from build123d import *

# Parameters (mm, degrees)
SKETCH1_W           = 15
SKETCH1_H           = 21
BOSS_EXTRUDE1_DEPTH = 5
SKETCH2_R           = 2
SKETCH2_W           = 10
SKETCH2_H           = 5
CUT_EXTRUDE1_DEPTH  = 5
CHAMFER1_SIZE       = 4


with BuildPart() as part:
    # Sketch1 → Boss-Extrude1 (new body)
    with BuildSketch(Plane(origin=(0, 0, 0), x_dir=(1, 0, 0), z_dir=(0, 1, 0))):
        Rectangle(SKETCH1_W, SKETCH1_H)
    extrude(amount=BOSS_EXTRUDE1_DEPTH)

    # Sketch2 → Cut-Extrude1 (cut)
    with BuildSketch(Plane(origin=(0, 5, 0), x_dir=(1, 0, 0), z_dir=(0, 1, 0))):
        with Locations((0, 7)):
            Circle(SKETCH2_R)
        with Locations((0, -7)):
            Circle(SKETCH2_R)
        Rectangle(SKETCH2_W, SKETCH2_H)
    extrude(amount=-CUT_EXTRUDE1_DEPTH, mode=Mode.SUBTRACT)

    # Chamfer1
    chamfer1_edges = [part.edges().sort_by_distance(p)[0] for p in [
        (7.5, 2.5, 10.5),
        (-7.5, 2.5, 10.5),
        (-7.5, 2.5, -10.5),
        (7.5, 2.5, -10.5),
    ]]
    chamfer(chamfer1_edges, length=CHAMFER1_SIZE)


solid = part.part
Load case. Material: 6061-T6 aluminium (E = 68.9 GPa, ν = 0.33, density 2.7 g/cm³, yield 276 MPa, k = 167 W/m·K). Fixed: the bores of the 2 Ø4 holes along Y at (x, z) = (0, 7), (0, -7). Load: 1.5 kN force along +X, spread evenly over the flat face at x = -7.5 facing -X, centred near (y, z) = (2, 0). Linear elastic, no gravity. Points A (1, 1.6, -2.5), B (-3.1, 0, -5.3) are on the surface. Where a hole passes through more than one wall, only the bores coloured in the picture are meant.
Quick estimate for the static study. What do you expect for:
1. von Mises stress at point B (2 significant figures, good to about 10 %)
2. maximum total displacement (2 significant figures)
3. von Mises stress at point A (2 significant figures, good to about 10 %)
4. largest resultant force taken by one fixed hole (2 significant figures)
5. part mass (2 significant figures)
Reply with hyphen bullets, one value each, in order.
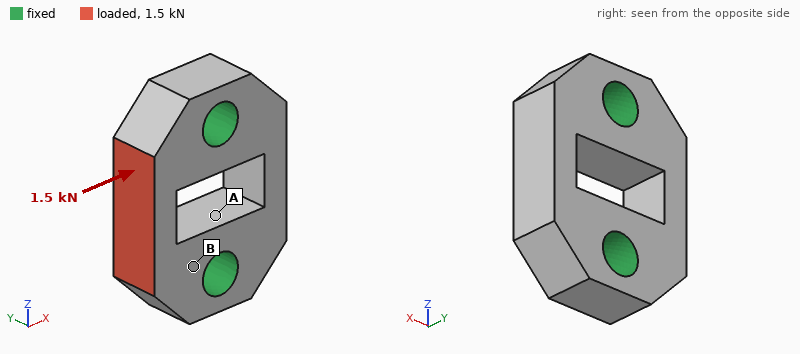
- 38 MPa
- 7.4 µm
- 11 MPa
- 790 N
- 2.8 g
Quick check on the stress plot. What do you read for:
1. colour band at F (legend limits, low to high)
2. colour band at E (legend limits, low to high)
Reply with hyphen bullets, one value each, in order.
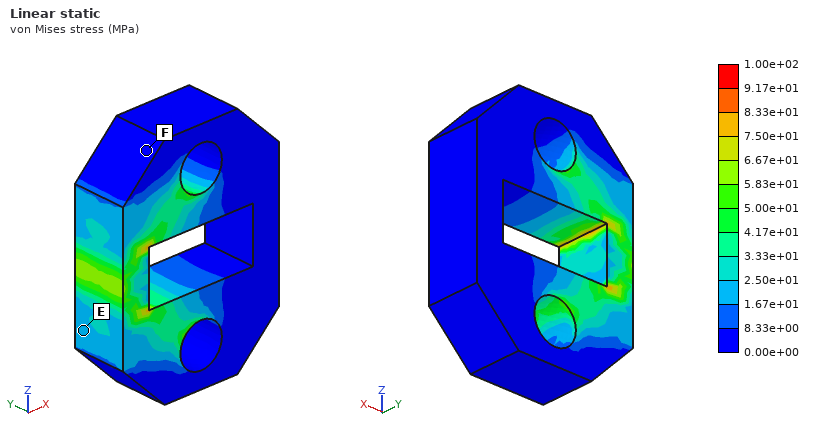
- 0.00e+00 to 8.33e+00 MPa
- 1.67e+01 to 2.50e+01 MPa
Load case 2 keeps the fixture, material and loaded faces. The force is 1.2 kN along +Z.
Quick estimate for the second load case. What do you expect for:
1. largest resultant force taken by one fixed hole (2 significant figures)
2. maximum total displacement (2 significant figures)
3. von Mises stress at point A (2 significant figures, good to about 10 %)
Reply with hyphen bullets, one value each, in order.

- 650 N
- 7.5 µm
- 15 MPa
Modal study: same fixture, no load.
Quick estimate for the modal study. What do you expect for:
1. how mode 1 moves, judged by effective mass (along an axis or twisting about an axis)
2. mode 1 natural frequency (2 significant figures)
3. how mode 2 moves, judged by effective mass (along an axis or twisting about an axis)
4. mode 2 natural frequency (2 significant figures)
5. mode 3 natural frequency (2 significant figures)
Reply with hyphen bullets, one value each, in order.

- twisting about Z
- 63 kHz
- along Y
- 66 kHz
- 79 kHz
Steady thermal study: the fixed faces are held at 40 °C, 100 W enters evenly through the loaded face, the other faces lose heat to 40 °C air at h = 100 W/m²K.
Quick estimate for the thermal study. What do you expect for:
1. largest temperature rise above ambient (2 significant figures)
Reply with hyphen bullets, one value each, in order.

- 83 K
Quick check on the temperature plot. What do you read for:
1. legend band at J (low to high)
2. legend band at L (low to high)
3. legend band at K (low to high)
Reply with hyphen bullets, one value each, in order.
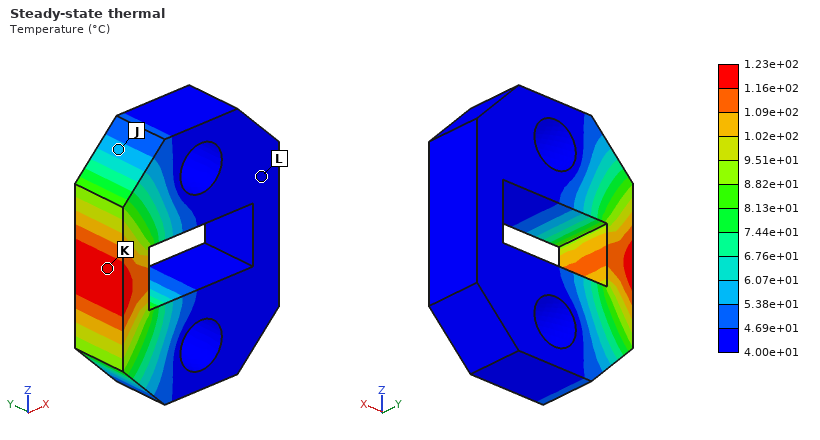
- 5.38e+01 to 6.07e+01 °C
- 4.00e+01 to 4.69e+01 °C
- 1.16e+02 to 1.23e+02 °C
